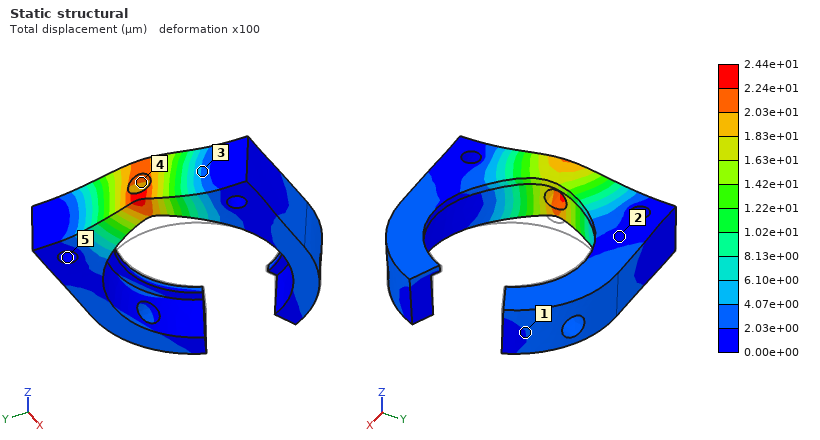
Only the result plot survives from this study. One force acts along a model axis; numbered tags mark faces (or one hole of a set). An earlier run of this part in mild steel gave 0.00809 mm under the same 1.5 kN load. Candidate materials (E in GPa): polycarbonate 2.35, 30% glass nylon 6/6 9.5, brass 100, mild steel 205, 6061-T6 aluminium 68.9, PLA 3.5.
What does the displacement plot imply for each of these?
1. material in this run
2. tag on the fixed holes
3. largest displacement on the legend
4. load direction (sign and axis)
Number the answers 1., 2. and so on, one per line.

1. 6061-T6 aluminium
2. 5
3. 2.44e+01 µm
4. +Z
